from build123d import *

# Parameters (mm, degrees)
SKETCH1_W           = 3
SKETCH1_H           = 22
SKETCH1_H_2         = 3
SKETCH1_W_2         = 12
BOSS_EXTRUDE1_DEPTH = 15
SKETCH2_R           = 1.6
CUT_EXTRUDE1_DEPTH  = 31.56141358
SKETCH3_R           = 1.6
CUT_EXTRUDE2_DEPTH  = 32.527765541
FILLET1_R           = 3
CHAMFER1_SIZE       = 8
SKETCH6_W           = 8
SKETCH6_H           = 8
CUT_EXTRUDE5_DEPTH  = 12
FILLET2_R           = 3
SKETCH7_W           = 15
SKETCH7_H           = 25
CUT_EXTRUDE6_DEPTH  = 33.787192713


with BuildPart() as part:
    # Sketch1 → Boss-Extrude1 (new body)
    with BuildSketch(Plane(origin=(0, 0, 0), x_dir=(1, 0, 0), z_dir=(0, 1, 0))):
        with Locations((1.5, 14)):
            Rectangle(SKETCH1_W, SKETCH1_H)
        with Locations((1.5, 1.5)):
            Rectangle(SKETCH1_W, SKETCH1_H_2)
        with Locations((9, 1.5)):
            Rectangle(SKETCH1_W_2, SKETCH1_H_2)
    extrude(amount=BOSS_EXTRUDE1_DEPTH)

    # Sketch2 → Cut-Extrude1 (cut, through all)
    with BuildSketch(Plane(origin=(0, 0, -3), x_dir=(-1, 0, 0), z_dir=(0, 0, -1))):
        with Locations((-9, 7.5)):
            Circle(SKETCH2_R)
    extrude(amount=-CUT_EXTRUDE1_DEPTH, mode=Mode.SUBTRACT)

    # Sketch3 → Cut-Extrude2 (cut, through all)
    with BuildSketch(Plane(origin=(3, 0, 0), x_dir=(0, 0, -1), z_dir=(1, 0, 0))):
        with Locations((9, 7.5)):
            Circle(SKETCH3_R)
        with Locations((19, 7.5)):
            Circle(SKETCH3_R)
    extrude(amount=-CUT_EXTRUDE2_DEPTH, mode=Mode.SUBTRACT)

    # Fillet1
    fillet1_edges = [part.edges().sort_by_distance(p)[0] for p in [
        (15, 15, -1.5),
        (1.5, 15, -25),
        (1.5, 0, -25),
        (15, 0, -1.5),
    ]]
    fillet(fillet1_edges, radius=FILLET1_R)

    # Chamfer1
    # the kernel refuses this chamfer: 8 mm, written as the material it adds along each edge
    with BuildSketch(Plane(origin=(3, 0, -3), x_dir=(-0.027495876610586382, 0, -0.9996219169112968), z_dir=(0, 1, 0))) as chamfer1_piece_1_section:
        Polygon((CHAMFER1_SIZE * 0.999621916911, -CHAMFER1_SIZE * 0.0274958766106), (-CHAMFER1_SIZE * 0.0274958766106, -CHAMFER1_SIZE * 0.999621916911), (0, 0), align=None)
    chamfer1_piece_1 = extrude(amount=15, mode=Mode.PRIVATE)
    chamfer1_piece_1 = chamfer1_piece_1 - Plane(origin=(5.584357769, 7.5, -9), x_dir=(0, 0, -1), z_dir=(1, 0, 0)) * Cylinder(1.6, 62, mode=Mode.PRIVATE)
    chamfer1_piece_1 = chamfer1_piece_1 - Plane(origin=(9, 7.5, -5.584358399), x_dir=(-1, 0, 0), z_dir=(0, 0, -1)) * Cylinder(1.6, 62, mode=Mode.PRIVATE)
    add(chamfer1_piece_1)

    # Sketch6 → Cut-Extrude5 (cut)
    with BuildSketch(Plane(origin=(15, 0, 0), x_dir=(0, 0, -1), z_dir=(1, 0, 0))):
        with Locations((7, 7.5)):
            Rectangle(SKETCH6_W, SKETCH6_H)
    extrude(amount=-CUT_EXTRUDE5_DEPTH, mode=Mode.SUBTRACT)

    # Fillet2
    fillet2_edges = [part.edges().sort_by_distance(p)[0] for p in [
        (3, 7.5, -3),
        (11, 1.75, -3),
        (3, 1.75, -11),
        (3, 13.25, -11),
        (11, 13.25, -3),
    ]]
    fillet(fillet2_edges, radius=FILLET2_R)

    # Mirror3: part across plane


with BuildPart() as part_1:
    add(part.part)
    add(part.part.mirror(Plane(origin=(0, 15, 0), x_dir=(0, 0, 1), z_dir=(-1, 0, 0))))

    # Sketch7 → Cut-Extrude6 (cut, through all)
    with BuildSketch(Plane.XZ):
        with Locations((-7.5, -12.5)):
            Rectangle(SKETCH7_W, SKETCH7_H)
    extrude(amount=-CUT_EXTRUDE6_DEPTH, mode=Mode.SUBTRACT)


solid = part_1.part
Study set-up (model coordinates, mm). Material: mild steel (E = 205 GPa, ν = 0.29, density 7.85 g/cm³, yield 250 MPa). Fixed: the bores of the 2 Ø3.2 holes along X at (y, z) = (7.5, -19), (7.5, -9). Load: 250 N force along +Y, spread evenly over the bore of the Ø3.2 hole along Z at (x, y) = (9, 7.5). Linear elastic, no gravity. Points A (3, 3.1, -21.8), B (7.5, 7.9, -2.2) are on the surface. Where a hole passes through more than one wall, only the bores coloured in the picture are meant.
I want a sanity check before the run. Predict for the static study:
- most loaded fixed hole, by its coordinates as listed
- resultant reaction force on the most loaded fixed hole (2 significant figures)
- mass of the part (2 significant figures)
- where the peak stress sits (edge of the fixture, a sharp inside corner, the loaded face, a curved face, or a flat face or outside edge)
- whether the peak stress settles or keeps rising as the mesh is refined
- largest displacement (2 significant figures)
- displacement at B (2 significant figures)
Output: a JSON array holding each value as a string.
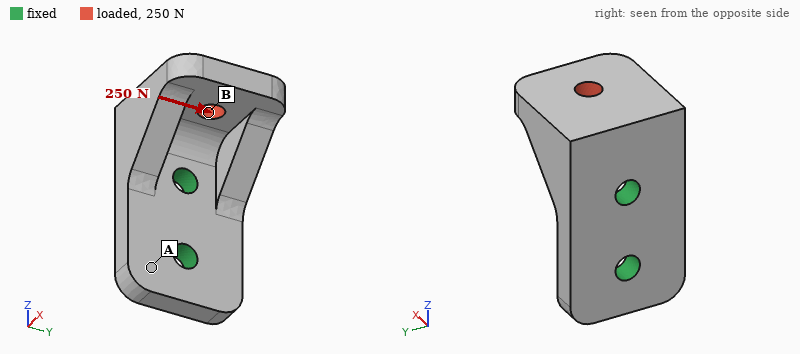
["(7.5, -9)", "370 N", "14 g", "edge of the fixture", "keeps rising", "9.9 µm", "4.6 µm"]
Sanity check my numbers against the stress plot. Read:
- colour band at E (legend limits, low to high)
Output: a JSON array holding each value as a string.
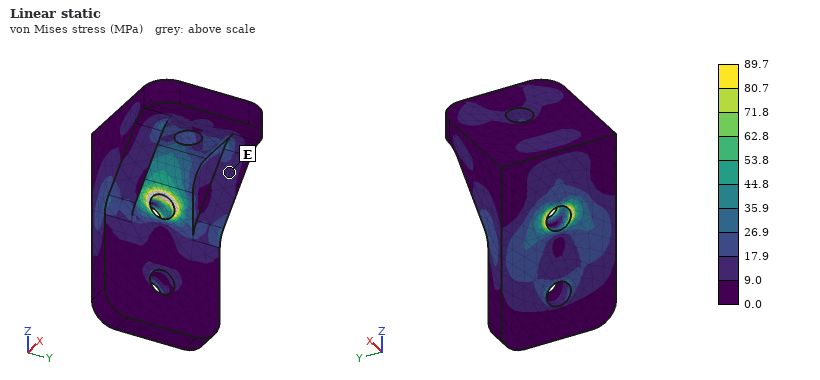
["9.0 to 17.9 MPa"]
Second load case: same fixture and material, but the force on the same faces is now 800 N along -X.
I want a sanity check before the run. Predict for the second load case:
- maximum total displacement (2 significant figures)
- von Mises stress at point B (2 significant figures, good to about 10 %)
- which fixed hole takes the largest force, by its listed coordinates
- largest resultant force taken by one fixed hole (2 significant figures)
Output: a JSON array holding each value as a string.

["26 µm", "37 MPa", "(7.5, -9)", "1.0 kN"]
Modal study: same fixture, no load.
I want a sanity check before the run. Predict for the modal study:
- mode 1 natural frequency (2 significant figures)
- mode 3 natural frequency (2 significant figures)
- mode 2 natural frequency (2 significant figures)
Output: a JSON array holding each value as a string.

["12 kHz", "29 kHz", "12 kHz"]
